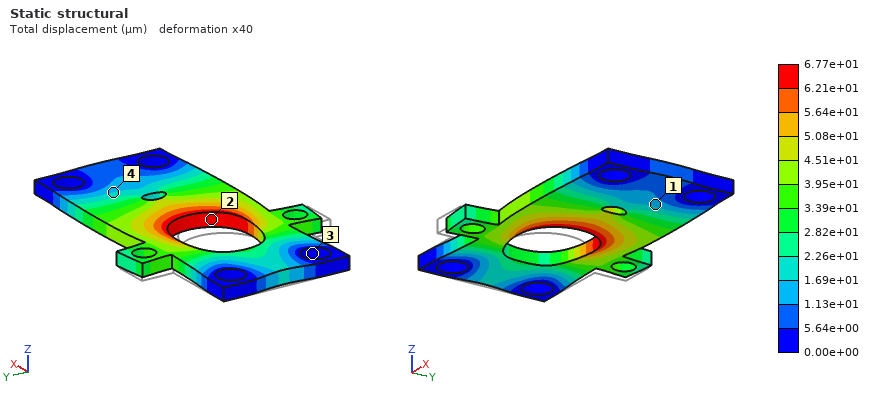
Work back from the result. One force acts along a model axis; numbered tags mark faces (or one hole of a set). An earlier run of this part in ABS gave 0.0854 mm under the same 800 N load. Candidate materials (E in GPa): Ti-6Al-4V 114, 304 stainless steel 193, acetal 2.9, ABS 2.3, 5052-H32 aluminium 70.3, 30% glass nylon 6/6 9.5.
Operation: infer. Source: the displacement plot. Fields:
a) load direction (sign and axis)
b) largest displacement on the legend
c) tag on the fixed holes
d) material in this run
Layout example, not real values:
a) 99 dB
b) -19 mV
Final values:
a) +X
b) 6.77e+01 µm
c) 3
d) acetal
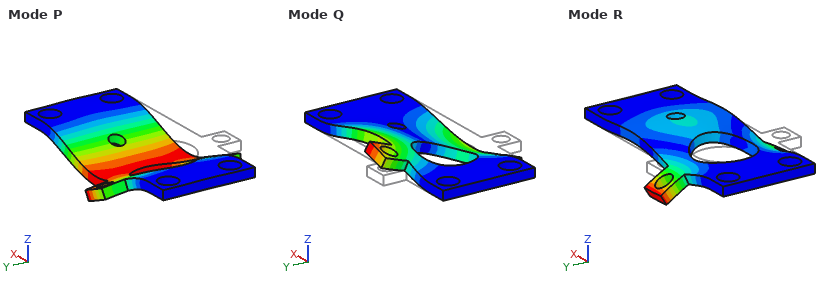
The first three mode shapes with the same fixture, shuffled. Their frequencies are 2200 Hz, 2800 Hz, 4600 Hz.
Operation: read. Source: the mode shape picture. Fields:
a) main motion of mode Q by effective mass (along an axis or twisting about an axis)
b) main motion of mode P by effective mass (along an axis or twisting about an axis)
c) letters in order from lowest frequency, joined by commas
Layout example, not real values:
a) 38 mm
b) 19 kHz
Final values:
a) twisting about X
b) along Z
c) P, Q, R
